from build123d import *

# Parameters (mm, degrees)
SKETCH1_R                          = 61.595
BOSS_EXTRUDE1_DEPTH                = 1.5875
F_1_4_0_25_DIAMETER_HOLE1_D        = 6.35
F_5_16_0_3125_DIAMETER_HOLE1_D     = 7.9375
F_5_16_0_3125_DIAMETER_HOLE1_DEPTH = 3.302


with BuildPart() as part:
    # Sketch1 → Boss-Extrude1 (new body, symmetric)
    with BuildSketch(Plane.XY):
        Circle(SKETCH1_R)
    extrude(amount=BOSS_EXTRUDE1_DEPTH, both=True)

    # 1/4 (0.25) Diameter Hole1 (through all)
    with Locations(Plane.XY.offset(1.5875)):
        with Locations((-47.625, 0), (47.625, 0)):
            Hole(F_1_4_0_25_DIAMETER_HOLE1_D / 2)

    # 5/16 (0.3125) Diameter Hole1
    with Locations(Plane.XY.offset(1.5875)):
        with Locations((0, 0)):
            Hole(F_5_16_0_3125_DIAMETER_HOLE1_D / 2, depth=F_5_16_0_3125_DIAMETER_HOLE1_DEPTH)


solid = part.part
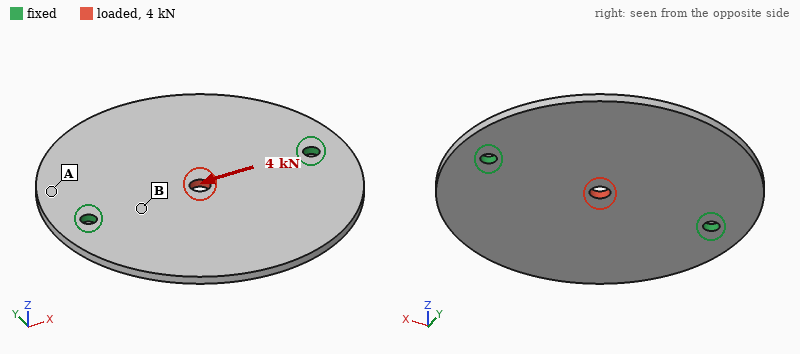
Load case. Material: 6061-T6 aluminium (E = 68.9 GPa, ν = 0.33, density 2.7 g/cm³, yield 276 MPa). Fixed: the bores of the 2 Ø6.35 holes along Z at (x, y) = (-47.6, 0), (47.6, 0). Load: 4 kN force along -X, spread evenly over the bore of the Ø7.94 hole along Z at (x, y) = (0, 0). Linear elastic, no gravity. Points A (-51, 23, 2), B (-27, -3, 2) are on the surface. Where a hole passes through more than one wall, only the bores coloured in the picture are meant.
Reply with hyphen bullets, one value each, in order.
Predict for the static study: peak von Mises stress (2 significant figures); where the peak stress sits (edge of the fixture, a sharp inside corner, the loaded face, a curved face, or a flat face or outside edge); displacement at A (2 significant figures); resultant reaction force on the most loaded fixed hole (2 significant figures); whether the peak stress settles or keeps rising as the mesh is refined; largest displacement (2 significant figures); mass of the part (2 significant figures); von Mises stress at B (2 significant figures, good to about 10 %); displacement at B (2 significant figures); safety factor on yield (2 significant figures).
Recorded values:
- 88 MPa
- the loaded face
- 6.7 µm
- 2.0 kN
- settles
- 18 µm
- 100 g
- 23 MPa
- 7.6 µm
- 3.1
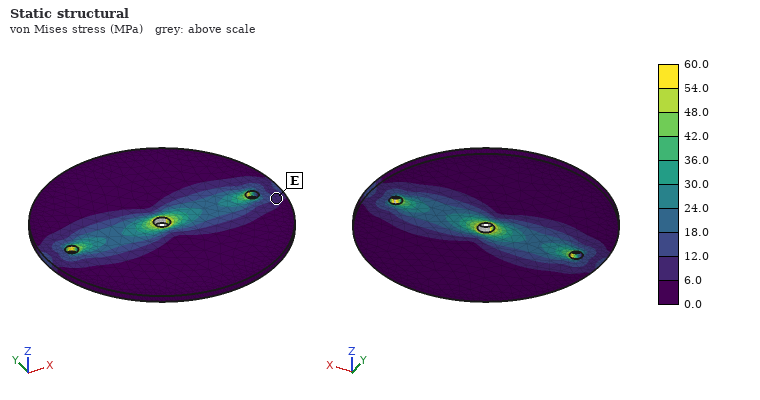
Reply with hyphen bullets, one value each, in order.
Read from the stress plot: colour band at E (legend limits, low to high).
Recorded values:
- 6.0 to 12.0 MPa
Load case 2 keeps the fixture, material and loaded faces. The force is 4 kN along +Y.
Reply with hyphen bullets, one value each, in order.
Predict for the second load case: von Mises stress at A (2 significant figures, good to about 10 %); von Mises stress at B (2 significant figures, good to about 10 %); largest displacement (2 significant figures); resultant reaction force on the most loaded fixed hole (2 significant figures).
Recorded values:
- 8.1 MPa
- 10 MPa
- 24 µm
- 2.0 kN
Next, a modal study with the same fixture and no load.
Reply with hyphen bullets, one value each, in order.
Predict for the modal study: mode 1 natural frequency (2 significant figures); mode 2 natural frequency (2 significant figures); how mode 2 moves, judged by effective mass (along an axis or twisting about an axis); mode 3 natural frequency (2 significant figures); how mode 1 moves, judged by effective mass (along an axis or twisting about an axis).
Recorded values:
- 620 Hz
- 810 Hz
- along Z
- 1800 Hz
- twisting about X
